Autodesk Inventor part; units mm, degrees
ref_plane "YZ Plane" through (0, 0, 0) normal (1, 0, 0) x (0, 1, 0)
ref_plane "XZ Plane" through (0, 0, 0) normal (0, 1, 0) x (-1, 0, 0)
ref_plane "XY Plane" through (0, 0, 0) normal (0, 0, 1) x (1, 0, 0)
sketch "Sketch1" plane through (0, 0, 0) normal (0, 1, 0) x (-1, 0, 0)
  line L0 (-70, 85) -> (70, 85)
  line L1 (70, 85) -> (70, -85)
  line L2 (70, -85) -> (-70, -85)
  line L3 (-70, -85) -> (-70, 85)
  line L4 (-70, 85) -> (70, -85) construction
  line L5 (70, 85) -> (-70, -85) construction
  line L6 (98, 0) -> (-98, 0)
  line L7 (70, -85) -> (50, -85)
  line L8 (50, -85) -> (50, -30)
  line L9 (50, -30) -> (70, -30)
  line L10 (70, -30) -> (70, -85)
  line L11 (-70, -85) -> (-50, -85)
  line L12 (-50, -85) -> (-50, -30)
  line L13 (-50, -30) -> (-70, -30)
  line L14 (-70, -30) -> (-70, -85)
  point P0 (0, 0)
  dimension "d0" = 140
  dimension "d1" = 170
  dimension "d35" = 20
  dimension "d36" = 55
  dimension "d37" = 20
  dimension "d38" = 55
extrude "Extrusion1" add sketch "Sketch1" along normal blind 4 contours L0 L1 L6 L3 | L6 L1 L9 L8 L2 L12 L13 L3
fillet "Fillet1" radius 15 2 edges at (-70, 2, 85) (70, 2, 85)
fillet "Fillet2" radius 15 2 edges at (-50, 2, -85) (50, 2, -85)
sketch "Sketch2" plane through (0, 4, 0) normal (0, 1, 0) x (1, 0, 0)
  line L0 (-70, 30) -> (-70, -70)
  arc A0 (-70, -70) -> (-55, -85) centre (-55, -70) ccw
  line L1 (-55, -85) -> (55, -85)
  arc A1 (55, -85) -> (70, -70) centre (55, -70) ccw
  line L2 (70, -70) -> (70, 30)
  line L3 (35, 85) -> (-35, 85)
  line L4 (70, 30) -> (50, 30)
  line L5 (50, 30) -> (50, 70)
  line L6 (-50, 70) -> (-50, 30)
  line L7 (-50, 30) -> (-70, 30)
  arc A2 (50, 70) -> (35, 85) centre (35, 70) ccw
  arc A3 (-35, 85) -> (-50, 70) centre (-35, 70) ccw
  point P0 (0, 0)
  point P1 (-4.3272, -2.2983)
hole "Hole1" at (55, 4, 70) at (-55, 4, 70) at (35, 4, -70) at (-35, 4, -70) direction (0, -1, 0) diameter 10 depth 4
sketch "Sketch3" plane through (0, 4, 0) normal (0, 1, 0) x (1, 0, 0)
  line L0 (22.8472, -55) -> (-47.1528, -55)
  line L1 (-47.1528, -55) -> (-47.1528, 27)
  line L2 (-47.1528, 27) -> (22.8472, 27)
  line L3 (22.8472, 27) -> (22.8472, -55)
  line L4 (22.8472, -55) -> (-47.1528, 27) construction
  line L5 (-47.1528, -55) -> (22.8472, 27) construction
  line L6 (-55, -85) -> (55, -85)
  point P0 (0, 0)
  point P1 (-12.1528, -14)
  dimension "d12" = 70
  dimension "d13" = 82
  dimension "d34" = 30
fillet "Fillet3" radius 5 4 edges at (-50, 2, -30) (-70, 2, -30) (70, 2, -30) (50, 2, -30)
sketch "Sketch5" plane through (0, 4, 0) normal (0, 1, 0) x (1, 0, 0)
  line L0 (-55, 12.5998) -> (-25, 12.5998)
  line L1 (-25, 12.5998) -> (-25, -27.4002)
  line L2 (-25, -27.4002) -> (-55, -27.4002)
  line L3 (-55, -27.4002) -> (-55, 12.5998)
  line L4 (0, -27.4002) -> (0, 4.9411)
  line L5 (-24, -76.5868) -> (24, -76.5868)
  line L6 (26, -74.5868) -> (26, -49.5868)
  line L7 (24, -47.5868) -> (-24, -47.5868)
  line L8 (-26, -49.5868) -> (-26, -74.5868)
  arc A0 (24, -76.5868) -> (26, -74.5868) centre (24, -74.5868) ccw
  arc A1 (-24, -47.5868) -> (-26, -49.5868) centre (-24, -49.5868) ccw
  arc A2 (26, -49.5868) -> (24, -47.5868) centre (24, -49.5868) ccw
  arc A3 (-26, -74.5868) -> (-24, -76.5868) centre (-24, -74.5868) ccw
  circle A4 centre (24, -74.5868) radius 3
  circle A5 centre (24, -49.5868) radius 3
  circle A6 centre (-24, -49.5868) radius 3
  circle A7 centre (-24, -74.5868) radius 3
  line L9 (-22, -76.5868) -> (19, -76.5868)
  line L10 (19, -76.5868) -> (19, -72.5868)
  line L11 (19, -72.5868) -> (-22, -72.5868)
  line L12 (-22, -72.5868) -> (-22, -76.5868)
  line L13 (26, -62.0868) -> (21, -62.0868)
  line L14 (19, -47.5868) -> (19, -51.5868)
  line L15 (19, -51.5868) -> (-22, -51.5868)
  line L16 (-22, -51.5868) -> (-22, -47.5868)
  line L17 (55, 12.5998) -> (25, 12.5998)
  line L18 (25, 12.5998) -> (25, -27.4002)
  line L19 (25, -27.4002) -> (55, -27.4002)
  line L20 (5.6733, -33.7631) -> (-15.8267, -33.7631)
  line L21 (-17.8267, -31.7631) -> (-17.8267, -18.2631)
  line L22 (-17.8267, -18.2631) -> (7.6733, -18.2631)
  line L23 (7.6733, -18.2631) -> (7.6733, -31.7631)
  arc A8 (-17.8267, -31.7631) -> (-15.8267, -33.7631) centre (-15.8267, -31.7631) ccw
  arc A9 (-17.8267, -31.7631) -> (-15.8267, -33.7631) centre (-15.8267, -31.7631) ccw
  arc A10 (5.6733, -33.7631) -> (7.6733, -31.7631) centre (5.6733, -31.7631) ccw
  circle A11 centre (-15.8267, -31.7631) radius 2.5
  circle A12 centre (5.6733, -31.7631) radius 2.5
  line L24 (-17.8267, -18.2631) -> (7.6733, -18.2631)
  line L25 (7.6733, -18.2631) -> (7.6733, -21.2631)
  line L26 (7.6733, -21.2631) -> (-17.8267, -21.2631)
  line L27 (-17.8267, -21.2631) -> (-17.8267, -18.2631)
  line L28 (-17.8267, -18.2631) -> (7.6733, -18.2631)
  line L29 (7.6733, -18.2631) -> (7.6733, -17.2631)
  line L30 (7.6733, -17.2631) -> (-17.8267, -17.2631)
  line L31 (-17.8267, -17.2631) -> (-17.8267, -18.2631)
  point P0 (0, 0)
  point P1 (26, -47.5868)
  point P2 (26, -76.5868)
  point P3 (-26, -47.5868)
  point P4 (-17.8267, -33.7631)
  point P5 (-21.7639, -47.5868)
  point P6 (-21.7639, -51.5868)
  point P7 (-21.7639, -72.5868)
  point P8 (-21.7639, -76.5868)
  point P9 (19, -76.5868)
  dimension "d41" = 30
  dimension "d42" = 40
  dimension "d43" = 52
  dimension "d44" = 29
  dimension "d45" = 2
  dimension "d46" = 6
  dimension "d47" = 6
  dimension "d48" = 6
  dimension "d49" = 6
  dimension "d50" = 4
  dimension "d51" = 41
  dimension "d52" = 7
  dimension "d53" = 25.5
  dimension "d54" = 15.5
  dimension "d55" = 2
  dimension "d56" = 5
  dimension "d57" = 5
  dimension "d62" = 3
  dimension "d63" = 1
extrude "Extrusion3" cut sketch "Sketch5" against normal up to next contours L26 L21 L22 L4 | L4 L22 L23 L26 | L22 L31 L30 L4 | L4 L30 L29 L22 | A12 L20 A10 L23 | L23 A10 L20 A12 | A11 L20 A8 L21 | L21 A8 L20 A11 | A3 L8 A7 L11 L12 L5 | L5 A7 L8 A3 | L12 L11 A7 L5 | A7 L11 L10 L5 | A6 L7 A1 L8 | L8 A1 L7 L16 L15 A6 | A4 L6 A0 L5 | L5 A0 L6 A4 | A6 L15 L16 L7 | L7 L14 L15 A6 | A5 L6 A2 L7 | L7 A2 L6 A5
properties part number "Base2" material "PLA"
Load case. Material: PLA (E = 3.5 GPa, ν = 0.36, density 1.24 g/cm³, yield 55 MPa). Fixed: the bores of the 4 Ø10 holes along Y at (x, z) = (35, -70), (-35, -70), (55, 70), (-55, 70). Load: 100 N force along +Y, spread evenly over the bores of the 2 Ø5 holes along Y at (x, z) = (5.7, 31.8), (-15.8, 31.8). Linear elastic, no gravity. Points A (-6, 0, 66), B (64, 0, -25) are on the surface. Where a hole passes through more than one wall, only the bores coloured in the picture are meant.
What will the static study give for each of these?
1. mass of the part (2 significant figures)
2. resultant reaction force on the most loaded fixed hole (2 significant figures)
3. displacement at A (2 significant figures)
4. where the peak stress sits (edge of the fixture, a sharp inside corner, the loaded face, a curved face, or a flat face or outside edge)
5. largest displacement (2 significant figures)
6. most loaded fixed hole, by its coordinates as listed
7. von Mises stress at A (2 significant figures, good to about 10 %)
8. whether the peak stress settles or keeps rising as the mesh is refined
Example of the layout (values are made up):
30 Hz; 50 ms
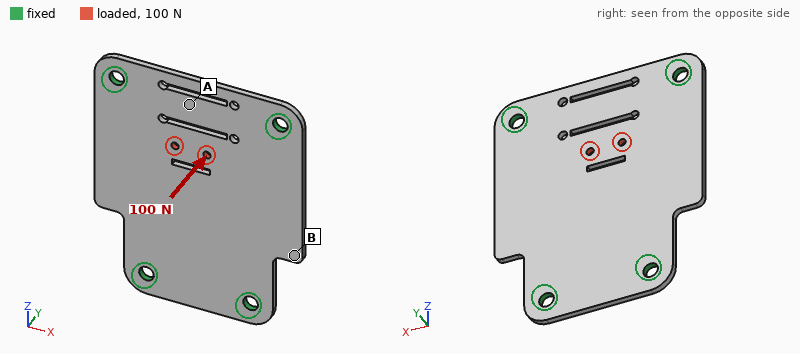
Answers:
100 g; 44 N; 0.31 mm; edge of the fixture; 0.97 mm; (-55, 70); 2.3 MPa; keeps rising
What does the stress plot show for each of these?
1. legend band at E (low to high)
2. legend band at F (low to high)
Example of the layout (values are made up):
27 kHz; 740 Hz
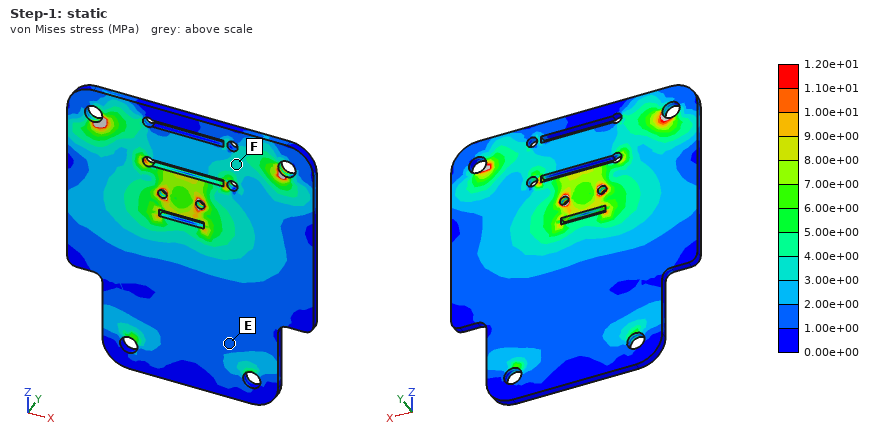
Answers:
1.00e+00 to 2.00e+00 MPa; 3.00e+00 to 4.00e+00 MPa
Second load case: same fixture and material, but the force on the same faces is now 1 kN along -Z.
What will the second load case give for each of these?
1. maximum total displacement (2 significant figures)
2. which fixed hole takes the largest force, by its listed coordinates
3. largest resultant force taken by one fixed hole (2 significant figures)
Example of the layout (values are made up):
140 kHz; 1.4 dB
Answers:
0.12 mm; (-55, 70); 340 N
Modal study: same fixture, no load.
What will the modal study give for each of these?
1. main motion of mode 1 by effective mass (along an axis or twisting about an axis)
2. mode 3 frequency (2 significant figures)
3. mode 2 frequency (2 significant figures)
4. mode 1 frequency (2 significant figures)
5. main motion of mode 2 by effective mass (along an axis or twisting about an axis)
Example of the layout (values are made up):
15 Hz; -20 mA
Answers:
along Y; 540 Hz; 390 Hz; 320 Hz; twisting about Z
